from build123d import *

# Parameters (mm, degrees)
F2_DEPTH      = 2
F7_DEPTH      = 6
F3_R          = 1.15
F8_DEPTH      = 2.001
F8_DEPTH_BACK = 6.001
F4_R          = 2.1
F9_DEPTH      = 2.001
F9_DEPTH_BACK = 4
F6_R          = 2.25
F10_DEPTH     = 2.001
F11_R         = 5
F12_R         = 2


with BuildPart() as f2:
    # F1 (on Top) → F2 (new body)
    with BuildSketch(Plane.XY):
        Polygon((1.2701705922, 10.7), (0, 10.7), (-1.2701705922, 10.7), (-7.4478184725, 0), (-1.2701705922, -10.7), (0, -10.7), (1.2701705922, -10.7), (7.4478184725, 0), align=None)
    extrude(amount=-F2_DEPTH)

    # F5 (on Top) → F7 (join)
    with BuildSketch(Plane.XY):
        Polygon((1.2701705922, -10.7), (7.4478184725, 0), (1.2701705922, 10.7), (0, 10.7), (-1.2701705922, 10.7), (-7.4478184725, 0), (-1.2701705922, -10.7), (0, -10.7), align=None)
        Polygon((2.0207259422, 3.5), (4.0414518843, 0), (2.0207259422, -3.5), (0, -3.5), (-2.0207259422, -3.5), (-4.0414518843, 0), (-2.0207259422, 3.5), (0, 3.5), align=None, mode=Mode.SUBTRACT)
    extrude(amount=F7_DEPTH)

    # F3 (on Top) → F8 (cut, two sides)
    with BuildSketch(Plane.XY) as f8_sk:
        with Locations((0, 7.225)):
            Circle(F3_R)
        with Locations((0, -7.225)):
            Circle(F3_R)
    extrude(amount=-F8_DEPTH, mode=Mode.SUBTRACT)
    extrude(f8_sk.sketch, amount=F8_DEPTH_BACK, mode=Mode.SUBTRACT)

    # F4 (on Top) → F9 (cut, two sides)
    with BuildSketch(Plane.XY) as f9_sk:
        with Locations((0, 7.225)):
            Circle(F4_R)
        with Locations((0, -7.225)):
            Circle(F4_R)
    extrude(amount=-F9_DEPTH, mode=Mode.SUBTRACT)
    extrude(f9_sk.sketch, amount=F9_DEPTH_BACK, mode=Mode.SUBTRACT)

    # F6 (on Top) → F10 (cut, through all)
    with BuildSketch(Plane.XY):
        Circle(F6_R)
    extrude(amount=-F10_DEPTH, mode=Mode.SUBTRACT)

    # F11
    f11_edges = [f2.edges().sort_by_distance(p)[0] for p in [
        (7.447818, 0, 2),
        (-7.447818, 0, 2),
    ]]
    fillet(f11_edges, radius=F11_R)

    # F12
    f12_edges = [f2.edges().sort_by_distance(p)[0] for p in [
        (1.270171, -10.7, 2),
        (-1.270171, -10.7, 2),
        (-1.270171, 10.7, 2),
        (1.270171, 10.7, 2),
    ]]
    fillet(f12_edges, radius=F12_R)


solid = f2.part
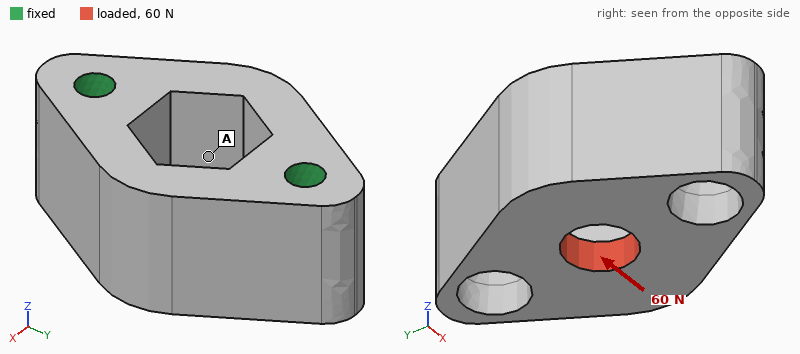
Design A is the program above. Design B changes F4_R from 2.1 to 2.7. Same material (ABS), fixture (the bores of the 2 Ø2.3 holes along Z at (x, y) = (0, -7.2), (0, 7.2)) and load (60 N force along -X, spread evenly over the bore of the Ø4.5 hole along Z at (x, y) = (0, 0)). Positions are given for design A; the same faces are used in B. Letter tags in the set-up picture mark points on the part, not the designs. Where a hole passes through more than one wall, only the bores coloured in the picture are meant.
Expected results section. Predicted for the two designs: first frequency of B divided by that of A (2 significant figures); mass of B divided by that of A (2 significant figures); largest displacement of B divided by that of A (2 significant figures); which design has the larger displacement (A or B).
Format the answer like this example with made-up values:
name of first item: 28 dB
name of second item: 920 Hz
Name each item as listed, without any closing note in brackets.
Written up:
first frequency of B divided by that of A: 0.92
mass of B divided by that of A: 0.89
largest displacement of B divided by that of A: 1.3
which design has the larger displacement: B
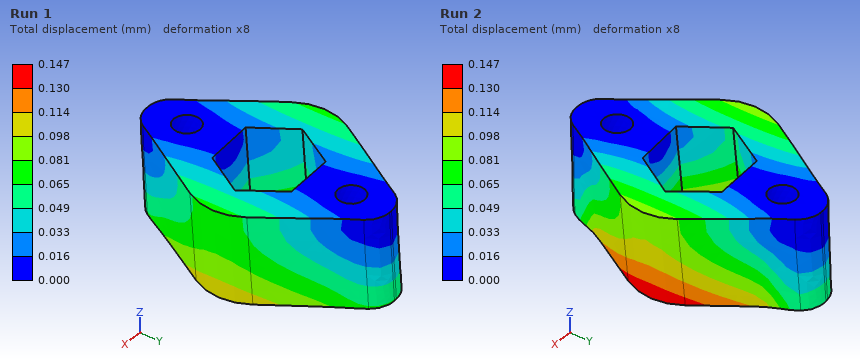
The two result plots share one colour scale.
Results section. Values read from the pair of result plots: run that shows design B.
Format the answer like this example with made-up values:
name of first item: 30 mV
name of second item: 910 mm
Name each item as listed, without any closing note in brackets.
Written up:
run that shows design B: Run 2
